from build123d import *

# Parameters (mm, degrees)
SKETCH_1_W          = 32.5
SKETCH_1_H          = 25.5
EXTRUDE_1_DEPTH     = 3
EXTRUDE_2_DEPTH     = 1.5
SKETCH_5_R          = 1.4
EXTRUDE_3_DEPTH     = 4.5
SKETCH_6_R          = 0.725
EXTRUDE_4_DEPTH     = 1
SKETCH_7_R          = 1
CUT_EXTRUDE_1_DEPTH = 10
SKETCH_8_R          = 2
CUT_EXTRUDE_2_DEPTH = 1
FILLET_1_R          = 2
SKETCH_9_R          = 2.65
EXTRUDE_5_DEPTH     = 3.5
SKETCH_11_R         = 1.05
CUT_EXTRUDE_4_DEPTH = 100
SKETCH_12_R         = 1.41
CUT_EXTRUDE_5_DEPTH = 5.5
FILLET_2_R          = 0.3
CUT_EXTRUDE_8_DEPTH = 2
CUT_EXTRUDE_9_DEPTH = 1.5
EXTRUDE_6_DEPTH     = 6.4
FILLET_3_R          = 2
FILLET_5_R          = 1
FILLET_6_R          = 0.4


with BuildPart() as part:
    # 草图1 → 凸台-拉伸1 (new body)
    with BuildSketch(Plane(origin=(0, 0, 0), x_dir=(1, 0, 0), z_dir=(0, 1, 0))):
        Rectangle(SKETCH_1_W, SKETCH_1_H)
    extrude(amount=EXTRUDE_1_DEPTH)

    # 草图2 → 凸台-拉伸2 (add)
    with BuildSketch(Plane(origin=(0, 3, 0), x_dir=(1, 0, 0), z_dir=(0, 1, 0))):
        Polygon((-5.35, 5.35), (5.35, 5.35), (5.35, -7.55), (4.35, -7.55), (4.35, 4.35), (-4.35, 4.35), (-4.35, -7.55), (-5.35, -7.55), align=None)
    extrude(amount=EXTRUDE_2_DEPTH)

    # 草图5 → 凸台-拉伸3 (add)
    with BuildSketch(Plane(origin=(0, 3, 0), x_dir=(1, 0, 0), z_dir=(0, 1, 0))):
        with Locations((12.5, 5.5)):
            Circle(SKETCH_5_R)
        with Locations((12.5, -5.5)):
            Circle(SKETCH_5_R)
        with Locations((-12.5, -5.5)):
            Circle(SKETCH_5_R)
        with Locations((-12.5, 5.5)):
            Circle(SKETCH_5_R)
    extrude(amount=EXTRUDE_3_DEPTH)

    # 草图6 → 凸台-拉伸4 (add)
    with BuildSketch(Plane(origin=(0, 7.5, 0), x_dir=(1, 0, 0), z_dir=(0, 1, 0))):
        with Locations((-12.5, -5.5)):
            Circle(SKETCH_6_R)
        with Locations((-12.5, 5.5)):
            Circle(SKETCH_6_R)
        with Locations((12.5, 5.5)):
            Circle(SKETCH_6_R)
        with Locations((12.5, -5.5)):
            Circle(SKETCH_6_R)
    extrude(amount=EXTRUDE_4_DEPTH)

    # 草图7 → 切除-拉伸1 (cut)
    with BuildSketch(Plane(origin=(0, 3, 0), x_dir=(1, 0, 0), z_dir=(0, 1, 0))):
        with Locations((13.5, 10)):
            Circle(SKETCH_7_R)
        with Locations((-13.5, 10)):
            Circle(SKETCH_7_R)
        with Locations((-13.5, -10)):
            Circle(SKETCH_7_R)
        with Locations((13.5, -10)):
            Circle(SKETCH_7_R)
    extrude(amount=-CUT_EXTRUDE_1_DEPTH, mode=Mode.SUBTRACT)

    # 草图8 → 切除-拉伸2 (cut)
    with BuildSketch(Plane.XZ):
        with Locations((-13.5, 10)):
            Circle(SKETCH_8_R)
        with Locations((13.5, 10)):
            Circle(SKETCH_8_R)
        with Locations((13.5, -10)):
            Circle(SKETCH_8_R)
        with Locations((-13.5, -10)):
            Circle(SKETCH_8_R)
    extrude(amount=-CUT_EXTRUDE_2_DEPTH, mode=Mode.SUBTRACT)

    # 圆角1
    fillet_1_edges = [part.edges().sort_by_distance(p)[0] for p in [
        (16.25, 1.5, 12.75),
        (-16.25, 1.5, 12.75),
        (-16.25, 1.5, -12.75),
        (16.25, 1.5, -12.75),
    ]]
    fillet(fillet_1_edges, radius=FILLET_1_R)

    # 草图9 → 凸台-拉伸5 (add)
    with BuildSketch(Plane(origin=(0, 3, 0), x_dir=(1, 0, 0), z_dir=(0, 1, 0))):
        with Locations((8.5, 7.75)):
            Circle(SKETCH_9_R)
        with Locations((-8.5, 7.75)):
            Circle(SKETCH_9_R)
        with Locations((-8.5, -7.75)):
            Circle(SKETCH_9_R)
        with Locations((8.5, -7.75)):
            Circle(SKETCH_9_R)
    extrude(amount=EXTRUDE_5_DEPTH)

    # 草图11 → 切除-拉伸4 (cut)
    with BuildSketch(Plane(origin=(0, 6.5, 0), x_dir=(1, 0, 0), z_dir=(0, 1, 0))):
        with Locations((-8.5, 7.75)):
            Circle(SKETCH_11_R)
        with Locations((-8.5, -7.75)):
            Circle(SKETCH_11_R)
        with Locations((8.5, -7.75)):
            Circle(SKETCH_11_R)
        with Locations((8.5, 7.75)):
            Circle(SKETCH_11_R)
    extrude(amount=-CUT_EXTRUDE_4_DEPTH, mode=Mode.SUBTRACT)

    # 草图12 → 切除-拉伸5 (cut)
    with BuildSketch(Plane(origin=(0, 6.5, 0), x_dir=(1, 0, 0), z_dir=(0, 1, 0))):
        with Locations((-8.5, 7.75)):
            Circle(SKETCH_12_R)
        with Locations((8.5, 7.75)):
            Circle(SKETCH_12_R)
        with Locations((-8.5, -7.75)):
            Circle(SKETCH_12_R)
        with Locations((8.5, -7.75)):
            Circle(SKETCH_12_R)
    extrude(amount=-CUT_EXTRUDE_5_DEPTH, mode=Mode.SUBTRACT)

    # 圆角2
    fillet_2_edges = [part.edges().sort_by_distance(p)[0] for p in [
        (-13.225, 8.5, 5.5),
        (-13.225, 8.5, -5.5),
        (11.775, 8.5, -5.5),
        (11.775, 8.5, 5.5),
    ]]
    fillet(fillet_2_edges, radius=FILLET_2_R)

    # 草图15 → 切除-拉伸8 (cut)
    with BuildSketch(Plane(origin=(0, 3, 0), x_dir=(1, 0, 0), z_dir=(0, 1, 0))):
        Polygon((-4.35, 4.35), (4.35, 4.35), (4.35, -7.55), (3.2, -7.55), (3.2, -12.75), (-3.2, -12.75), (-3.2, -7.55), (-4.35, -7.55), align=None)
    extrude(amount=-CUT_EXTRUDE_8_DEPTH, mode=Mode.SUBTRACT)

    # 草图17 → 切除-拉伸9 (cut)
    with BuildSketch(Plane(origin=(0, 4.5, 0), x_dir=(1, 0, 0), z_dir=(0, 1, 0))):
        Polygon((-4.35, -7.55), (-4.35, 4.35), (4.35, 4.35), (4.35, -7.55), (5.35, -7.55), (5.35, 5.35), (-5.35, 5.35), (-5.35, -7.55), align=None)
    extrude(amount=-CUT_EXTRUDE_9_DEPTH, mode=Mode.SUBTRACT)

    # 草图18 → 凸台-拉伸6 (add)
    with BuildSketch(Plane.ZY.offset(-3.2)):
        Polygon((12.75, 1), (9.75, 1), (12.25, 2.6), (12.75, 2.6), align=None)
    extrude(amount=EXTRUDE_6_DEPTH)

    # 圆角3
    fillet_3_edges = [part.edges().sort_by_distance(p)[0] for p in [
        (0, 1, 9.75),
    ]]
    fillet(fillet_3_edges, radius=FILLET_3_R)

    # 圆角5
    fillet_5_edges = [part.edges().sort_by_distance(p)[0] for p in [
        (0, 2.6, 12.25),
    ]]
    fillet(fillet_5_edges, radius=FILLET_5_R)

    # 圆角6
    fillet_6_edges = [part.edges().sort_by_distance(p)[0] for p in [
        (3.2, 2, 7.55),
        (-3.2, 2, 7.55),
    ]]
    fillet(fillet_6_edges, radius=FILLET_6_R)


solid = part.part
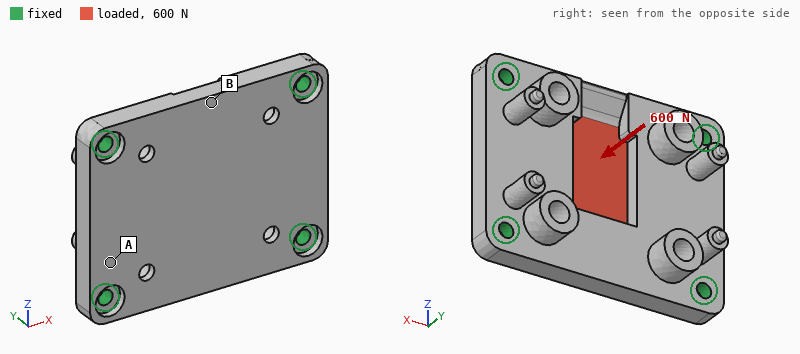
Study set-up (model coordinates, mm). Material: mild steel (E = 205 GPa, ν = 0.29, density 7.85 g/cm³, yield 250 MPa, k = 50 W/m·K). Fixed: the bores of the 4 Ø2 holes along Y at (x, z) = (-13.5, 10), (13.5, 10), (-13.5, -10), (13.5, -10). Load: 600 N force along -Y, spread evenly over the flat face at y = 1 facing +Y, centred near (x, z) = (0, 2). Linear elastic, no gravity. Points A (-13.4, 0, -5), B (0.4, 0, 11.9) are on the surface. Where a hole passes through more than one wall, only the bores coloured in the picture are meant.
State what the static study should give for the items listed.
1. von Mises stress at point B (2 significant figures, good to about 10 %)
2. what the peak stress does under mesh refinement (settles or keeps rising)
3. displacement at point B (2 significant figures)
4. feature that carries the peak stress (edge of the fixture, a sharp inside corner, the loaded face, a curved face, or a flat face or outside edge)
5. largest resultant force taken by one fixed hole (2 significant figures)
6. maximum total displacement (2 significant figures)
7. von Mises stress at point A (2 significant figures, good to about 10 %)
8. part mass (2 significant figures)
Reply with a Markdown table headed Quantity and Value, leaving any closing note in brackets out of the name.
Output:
| Quantity | Value |
|---|---|
| von Mises stress at point B | 76 MPa |
| what the peak stress does under mesh refinement | keeps rising |
| displacement at point B | 13 µm |
| feature that carries the peak stress | edge of the fixture |
| largest resultant force taken by one fixed hole | 470 N |
| maximum total displacement | 22 µm |
| von Mises stress at point A | 27 MPa |
| part mass | 19 g |
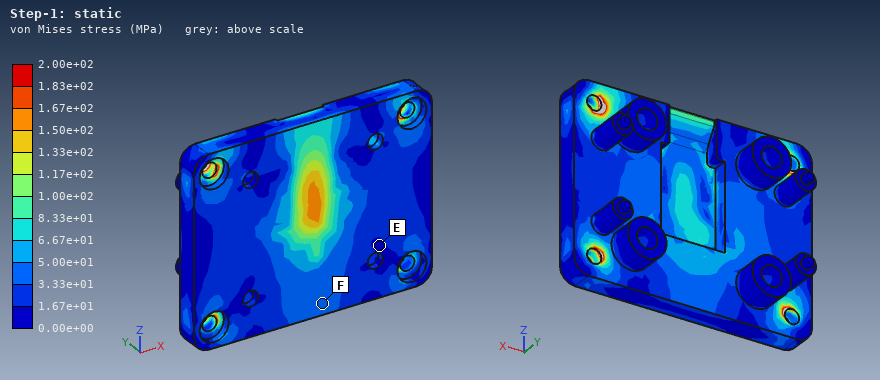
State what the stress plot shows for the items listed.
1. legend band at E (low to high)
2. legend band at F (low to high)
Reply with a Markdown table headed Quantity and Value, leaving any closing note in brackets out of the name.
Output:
| Quantity | Value |
|---|---|
| legend band at E | 0.00e+00 to 1.67e+01 MPa |
| legend band at F | 3.33e+01 to 5.00e+01 MPa |
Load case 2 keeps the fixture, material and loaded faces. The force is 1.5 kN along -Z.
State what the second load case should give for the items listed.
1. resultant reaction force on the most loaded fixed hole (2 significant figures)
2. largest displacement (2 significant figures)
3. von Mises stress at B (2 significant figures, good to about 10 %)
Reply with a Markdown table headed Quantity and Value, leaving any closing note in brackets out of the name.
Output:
| Quantity | Value |
|---|---|
| resultant reaction force on the most loaded fixed hole | 450 N |
| largest displacement | 3.7 µm |
| von Mises stress at B | 34 MPa |
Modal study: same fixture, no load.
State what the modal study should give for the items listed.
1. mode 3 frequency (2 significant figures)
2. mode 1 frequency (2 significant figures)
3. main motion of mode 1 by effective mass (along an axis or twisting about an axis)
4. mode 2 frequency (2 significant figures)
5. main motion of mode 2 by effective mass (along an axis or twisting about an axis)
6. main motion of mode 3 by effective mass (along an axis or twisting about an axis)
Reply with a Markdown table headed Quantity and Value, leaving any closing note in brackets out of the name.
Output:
| Quantity | Value |
|---|---|
| mode 3 frequency | 25 kHz |
| mode 1 frequency | 14 kHz |
| main motion of mode 1 by effective mass | along Y |
| mode 2 frequency | 21 kHz |
| main motion of mode 2 by effective mass | twisting about X |
| main motion of mode 3 by effective mass | twisting about Z |
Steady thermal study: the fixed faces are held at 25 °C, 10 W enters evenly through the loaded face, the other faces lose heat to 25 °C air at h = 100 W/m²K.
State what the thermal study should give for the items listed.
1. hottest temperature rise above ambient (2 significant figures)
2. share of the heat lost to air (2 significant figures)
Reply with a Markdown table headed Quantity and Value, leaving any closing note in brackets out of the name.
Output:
| Quantity | Value |
|---|---|
| hottest temperature rise above ambient | 33 K |
| share of the heat lost to air | 24 % |
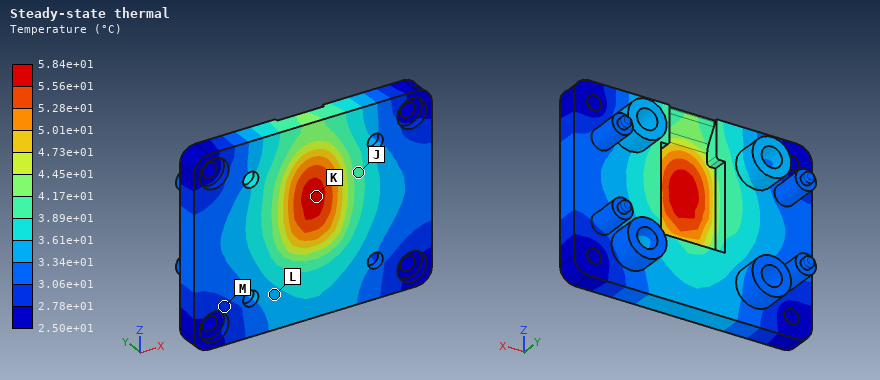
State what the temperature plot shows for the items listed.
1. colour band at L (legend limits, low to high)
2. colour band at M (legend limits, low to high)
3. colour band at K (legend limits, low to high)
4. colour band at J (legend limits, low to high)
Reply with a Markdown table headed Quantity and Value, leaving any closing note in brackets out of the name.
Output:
| Quantity | Value |
|---|---|
| colour band at L | 3.34e+01 to 3.61e+01 °C |
| colour band at M | 2.78e+01 to 3.06e+01 °C |
| colour band at K | 5.56e+01 to 5.84e+01 °C |
| colour band at J | 3.89e+01 to 4.17e+01 °C |
